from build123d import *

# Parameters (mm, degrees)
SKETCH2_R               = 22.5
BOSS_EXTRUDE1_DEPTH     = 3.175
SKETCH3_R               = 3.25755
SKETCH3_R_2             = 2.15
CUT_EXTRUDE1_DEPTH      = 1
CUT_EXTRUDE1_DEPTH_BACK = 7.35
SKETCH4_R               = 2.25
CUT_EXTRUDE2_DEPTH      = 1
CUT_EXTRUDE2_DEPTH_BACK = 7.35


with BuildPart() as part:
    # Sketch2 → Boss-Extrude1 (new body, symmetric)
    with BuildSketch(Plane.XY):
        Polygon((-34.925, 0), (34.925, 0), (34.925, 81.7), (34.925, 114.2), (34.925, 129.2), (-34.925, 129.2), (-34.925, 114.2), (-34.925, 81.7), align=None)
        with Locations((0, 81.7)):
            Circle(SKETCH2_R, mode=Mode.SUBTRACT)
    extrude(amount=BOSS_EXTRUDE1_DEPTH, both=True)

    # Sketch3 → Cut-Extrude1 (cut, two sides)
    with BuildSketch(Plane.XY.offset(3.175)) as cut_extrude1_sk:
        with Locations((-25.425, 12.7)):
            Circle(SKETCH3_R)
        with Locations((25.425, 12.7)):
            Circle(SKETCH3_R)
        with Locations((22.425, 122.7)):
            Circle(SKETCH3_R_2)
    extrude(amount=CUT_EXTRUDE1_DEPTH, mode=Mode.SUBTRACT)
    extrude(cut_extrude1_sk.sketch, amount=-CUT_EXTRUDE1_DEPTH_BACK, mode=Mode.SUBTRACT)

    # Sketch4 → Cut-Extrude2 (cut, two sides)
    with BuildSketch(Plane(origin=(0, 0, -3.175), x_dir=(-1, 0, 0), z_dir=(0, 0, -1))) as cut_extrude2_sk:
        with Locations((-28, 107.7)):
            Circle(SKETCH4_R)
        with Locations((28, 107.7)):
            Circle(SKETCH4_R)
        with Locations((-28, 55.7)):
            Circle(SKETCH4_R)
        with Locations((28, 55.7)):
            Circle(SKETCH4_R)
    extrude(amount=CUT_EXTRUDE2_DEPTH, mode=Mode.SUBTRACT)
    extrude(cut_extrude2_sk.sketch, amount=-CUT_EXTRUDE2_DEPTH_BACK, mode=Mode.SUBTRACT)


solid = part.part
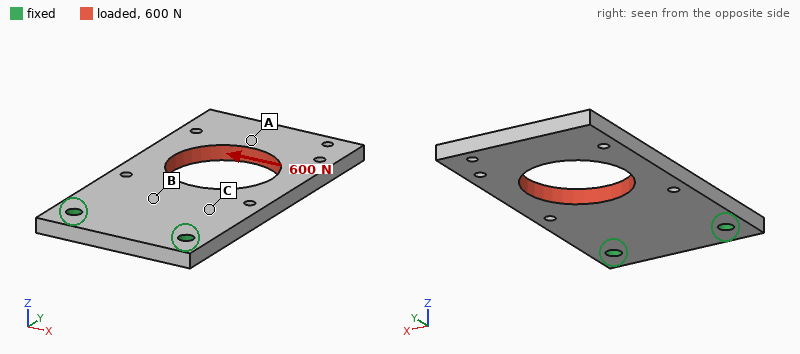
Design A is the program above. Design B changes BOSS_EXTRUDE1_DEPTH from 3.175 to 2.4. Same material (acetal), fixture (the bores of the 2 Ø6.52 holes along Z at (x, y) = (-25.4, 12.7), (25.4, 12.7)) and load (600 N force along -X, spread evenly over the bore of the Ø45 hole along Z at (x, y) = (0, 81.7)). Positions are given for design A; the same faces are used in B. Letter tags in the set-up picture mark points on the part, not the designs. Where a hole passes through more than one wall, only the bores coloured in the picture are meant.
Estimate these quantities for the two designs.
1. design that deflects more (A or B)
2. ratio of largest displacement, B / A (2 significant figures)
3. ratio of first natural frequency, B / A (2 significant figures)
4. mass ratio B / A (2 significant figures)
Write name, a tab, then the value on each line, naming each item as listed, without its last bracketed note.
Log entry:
design that deflects more	B
ratio of largest displacement, B / A	1.3
ratio of first natural frequency, B / A	0.76
mass ratio B / A	0.76
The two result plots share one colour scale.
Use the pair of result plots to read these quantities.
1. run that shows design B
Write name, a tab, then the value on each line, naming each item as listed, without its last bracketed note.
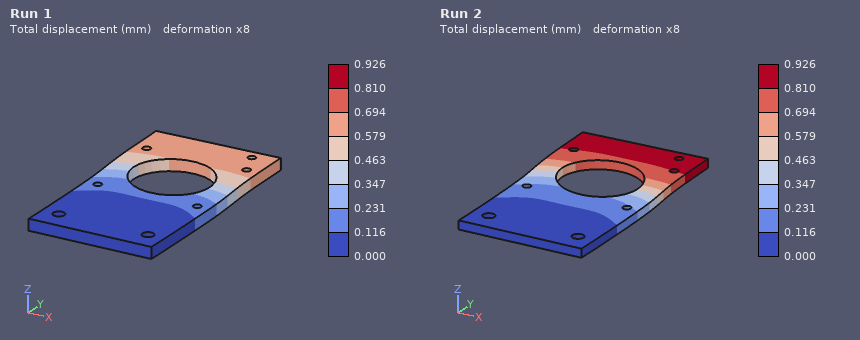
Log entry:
run that shows design B	Run 2
